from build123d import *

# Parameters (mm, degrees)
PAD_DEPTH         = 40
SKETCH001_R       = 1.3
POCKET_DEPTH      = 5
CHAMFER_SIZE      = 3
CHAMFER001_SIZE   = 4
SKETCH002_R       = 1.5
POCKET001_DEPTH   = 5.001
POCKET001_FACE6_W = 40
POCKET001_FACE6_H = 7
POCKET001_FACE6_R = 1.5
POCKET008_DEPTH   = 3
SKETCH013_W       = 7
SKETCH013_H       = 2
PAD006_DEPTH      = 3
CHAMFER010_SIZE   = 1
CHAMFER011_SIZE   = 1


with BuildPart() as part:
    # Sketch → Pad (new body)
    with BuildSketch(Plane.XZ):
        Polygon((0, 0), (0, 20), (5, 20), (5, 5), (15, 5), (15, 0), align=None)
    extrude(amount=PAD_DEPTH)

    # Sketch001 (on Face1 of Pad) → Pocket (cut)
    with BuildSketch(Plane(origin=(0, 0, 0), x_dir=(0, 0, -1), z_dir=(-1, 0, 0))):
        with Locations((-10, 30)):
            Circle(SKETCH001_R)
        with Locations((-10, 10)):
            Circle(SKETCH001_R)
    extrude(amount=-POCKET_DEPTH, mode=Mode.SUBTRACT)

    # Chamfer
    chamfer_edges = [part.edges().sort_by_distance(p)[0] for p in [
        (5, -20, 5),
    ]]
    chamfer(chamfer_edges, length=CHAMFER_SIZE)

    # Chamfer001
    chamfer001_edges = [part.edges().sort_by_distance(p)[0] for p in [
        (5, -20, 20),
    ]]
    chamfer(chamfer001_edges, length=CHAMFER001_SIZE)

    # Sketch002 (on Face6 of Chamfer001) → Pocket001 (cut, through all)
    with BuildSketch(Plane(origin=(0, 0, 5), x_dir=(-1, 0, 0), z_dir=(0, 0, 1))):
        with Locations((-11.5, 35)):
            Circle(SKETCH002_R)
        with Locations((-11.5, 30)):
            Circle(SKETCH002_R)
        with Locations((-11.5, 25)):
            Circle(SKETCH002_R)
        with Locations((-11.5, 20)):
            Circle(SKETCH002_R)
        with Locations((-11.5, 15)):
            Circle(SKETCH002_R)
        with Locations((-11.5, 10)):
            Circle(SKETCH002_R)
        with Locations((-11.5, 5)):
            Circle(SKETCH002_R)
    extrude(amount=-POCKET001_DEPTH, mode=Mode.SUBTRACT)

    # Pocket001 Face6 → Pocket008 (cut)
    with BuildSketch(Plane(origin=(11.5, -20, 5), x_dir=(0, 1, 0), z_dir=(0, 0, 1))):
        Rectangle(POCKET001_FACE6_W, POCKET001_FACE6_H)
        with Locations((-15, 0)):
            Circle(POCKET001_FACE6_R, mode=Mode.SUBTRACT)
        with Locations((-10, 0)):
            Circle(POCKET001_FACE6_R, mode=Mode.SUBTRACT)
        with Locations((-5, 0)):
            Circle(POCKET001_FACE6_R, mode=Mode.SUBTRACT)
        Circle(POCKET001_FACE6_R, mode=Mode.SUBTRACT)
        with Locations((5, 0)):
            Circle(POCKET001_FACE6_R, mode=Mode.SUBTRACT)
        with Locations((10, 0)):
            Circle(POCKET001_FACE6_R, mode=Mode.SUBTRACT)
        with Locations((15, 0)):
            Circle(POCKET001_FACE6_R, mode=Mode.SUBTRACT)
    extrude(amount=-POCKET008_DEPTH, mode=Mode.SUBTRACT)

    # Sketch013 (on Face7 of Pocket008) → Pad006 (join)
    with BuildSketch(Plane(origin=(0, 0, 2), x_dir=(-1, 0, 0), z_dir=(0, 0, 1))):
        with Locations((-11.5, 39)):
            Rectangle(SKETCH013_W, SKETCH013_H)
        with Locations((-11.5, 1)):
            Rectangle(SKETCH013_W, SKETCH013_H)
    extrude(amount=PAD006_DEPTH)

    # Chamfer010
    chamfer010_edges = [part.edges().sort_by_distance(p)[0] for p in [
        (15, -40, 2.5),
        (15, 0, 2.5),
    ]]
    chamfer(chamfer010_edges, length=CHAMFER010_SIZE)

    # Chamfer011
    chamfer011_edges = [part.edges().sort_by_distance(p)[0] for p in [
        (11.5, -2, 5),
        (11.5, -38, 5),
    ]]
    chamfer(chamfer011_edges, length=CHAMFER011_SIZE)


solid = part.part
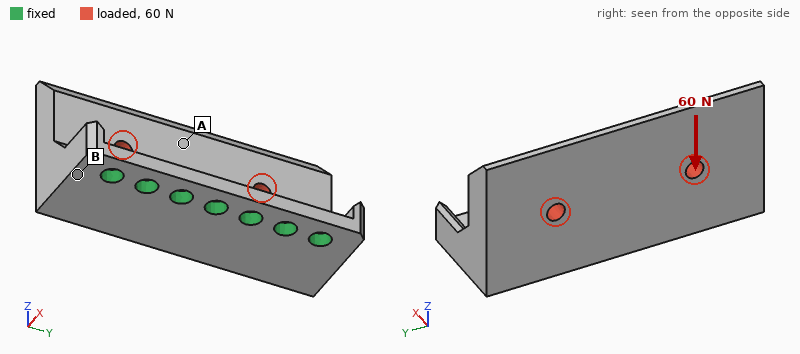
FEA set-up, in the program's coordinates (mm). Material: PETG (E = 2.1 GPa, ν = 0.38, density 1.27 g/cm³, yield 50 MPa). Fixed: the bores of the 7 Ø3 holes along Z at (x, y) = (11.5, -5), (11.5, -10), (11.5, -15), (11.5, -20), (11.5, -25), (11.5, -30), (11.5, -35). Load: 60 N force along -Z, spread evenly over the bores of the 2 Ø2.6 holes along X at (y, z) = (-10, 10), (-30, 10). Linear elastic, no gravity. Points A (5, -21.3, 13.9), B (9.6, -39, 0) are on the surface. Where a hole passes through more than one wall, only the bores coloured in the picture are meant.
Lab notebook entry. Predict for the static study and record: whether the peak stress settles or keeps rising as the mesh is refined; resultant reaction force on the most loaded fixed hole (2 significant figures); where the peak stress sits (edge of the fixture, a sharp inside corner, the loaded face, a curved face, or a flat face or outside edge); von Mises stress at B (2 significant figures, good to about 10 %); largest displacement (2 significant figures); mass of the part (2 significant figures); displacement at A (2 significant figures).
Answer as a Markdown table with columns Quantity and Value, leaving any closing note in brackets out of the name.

| Quantity | Value |
|---|---|
| whether the peak stress settles or keeps rising as the mesh is refined | keeps rising |
| resultant reaction force on the most loaded fixed hole | 12 N |
| where the peak stress sits | edge of the fixture |
| von Mises stress at B | 5.1 MPa |
| largest displacement | 0.34 mm |
| mass of the part | 6.3 g |
| displacement at A | 0.22 mm |
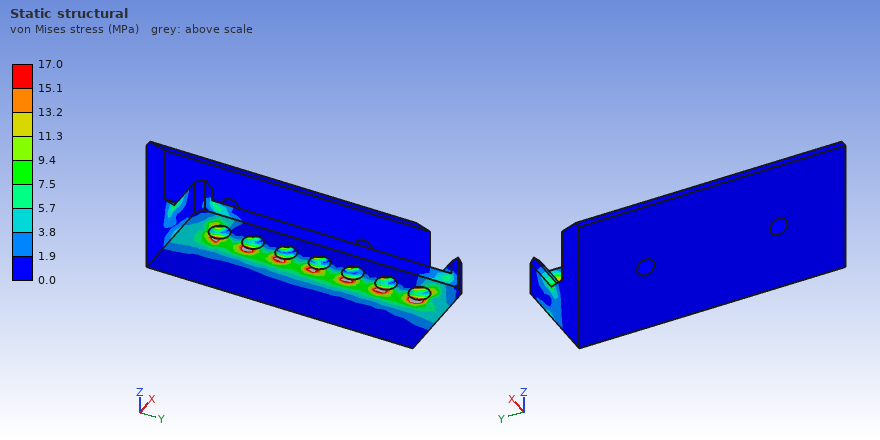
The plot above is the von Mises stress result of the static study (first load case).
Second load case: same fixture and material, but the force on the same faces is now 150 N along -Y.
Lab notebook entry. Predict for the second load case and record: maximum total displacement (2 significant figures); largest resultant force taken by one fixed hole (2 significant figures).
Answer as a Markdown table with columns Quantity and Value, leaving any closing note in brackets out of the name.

| Quantity | Value |
|---|---|
| maximum total displacement | 0.10 mm |
| largest resultant force taken by one fixed hole | 49 N |
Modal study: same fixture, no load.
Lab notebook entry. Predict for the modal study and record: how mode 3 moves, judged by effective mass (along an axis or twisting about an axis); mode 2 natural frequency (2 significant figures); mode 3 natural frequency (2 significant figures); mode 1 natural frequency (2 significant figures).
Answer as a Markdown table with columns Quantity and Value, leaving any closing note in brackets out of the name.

| Quantity | Value |
|---|---|
| how mode 3 moves, judged by effective mass | along Y |
| mode 2 natural frequency | 2500 Hz |
| mode 3 natural frequency | 4800 Hz |
| mode 1 natural frequency | 950 Hz |
